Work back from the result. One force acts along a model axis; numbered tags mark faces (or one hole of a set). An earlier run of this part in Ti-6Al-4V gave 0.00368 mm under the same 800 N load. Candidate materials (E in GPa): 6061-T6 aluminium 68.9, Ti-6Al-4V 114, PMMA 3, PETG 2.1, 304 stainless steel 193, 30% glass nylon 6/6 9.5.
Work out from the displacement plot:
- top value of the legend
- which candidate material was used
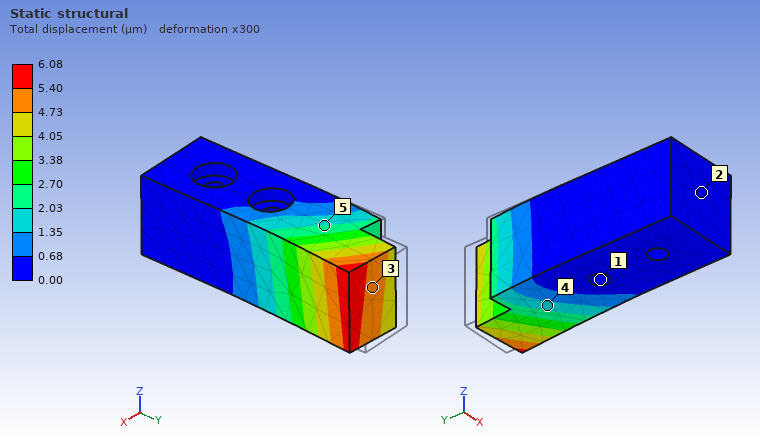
6.08 µm
6061-T6 aluminium
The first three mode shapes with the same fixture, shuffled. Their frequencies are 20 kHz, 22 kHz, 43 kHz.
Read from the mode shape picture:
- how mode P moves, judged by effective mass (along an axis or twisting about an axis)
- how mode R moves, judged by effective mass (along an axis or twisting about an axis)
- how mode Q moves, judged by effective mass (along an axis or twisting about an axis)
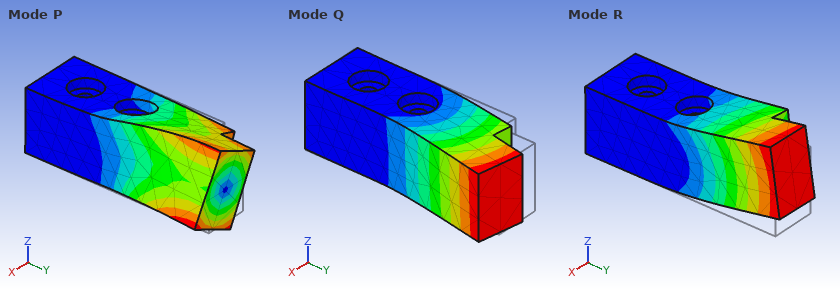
twisting about Y
along Z
along X
